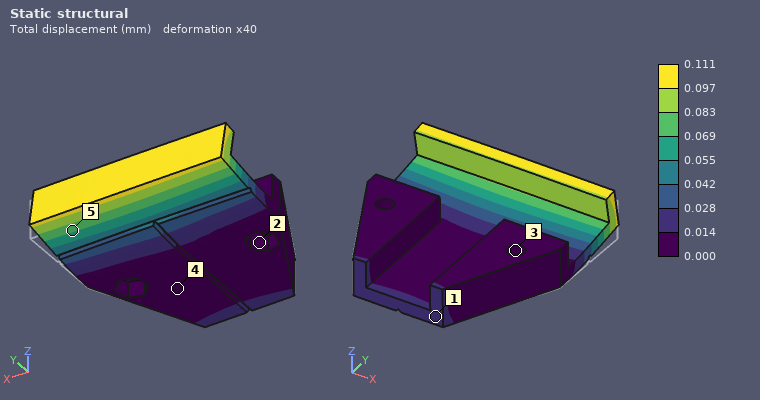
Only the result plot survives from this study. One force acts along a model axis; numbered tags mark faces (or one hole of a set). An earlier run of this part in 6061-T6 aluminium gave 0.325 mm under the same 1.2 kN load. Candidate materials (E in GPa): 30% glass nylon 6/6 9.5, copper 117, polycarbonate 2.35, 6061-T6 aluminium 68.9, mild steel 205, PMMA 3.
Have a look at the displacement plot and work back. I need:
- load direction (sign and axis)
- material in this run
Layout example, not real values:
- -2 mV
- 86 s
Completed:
- +Z
- mild steel
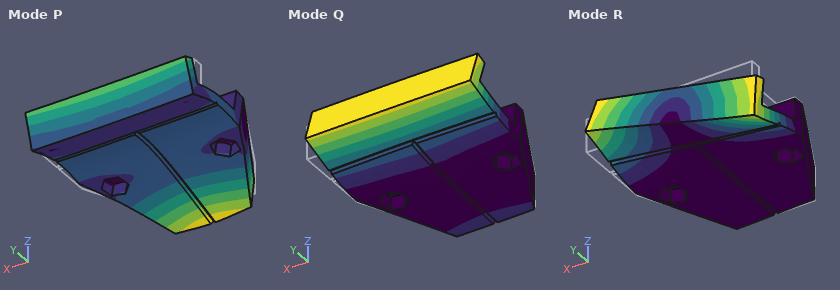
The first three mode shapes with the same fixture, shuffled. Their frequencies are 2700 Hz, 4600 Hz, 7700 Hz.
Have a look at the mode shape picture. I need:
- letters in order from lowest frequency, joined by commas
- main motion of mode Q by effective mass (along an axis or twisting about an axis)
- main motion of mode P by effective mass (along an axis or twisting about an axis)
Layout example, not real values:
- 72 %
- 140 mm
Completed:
- Q, R, P
- along Z
- along Y
